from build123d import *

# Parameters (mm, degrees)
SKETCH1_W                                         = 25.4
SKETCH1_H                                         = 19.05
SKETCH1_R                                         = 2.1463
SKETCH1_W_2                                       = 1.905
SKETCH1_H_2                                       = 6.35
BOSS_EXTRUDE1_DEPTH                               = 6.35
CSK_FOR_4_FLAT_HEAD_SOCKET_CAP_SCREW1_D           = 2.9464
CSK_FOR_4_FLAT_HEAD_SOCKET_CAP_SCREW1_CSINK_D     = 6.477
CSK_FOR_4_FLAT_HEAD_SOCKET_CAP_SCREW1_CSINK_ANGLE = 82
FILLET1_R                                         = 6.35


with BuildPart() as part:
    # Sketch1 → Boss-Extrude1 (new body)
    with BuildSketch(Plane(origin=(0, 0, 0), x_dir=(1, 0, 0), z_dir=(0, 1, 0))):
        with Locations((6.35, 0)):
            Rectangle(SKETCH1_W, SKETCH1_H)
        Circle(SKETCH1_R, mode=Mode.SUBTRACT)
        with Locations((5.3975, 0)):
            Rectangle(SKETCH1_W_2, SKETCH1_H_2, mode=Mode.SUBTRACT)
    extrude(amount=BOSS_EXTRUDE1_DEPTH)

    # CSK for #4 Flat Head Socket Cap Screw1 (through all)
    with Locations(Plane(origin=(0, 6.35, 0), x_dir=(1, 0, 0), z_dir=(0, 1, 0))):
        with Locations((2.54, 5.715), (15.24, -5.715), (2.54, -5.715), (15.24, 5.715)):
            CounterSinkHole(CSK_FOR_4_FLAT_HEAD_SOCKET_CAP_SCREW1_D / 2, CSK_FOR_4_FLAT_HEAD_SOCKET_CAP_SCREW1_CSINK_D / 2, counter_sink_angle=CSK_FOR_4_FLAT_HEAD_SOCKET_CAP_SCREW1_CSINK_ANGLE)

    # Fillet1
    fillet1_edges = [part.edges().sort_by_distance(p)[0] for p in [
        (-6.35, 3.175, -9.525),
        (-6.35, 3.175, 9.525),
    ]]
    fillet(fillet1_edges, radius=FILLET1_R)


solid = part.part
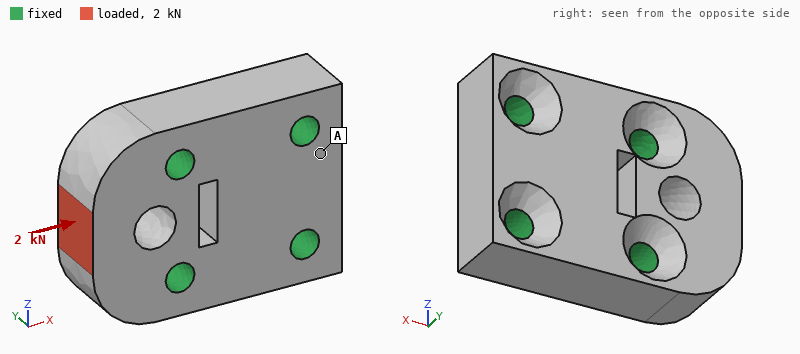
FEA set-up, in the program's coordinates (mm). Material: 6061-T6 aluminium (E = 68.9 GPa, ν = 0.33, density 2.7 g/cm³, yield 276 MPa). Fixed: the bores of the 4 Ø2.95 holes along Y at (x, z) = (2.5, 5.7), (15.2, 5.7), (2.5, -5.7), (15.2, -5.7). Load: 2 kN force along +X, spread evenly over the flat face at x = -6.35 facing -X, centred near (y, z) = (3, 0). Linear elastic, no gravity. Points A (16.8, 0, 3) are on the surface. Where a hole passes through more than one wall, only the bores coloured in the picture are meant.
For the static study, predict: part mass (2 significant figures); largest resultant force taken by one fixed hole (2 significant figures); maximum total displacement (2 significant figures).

6.8 g
1.0 kN
10 µm
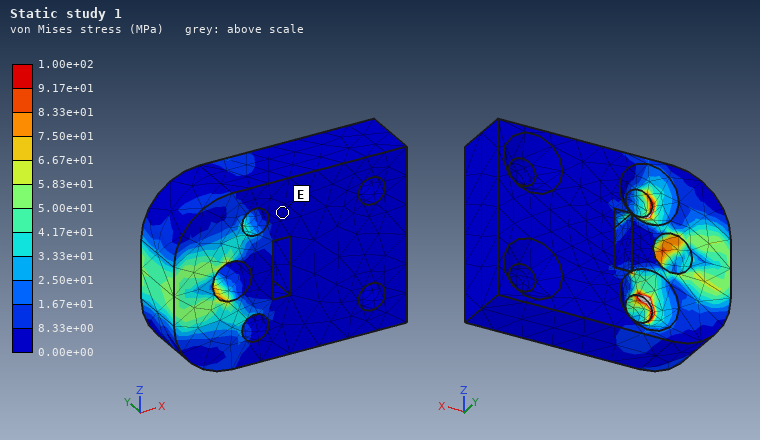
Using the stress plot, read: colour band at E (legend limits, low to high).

0.00e+00 to 8.33e+00 MPa
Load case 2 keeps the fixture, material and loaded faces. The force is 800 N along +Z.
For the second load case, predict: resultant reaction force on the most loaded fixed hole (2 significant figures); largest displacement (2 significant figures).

580 N
5.0 µm
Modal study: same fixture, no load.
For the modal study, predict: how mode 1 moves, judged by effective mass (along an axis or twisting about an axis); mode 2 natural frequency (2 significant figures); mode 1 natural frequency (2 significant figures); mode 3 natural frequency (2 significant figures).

along Y
68 kHz
42 kHz
70 kHz
